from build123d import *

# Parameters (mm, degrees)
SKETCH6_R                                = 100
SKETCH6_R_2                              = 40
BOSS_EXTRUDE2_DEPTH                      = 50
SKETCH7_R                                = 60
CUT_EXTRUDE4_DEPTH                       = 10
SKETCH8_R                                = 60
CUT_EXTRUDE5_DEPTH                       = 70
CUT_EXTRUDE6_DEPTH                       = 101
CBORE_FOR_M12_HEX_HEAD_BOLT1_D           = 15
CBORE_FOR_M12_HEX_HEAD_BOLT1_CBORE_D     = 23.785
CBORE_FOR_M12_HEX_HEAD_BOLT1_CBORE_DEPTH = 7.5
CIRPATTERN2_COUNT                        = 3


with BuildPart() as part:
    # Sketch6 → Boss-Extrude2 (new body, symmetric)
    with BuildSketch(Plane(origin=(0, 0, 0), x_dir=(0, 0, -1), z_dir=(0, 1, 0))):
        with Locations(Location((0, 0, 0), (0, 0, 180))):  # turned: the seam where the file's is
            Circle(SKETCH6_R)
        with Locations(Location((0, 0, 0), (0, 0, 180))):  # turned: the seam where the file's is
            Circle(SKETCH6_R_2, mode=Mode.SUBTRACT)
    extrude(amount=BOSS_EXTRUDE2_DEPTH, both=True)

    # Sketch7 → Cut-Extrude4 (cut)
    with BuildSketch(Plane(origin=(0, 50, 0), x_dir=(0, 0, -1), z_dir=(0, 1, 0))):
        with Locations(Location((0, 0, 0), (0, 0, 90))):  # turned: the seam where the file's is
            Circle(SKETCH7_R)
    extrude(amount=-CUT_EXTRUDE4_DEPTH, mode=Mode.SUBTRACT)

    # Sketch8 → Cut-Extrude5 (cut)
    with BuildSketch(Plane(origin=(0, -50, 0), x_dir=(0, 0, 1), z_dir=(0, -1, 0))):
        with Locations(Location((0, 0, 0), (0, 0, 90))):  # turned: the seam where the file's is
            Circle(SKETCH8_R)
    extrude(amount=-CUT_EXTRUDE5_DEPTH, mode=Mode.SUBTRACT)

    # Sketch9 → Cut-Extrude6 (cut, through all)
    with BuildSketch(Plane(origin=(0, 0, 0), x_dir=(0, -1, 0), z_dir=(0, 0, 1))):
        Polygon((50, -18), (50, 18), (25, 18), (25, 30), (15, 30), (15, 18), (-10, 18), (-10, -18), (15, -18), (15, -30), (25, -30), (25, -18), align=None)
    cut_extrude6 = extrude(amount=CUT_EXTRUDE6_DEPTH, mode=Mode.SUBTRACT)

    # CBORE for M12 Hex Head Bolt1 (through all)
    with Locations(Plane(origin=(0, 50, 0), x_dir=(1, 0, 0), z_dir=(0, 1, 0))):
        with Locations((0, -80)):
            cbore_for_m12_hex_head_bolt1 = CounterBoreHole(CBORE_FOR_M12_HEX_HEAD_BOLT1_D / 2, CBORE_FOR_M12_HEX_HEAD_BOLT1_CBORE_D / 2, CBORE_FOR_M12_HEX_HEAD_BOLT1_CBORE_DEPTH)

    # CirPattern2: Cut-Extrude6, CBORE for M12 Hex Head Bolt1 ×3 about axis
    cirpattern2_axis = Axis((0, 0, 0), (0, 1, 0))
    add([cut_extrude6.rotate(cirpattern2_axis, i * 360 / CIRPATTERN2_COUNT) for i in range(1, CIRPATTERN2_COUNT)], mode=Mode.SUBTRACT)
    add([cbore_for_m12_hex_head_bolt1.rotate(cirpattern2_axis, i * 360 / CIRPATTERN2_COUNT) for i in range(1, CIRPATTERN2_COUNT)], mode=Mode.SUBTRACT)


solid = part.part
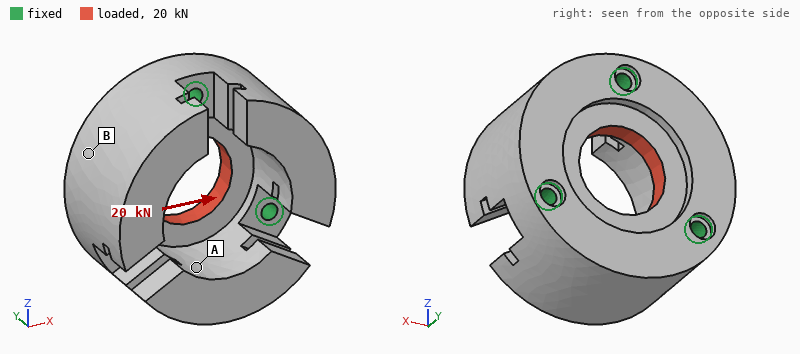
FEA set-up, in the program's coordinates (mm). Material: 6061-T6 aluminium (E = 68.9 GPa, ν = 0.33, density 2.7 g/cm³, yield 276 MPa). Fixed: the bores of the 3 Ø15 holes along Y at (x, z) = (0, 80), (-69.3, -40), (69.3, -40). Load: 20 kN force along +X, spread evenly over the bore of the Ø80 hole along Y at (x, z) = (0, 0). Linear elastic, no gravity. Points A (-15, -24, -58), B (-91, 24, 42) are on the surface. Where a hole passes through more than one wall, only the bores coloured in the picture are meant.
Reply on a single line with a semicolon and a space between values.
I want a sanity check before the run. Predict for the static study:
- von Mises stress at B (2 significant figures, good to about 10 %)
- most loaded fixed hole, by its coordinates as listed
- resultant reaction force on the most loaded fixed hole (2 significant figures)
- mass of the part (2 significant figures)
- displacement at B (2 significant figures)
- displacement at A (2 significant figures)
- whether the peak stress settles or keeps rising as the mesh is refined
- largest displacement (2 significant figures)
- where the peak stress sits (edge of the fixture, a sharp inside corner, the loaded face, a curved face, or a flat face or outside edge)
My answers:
1.9 MPa; (0, 80); 7.8 kN; 4.9 kg; 3.3 µm; 1.0 µm; keeps rising; 5.5 µm; edge of the fixture
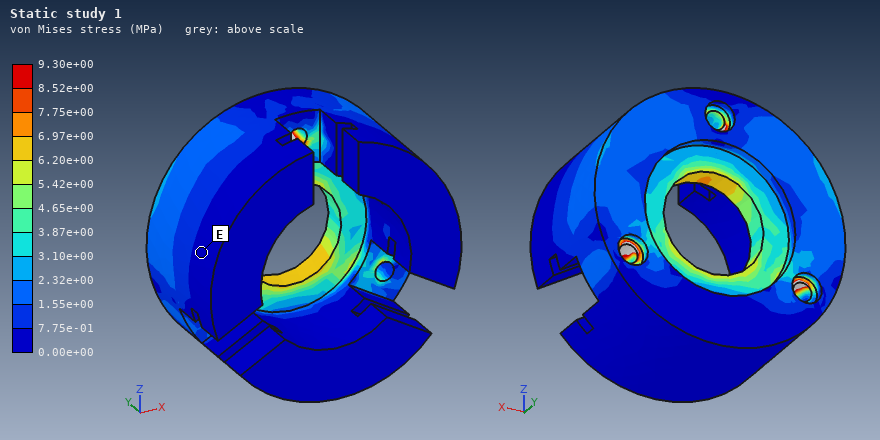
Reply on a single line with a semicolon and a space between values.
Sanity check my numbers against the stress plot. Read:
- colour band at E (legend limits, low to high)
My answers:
0.00e+00 to 7.75e-01 MPa
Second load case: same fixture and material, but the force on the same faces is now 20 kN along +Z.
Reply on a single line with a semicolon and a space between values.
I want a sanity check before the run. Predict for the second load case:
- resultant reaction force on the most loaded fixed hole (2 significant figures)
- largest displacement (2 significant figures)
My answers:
7.3 kN; 6.2 µm
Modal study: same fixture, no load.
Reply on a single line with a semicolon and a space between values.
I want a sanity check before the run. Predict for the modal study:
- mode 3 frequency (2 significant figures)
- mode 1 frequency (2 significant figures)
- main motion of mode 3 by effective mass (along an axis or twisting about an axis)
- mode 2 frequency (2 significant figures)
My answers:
2200 Hz; 2100 Hz; along Y; 2100 Hz
